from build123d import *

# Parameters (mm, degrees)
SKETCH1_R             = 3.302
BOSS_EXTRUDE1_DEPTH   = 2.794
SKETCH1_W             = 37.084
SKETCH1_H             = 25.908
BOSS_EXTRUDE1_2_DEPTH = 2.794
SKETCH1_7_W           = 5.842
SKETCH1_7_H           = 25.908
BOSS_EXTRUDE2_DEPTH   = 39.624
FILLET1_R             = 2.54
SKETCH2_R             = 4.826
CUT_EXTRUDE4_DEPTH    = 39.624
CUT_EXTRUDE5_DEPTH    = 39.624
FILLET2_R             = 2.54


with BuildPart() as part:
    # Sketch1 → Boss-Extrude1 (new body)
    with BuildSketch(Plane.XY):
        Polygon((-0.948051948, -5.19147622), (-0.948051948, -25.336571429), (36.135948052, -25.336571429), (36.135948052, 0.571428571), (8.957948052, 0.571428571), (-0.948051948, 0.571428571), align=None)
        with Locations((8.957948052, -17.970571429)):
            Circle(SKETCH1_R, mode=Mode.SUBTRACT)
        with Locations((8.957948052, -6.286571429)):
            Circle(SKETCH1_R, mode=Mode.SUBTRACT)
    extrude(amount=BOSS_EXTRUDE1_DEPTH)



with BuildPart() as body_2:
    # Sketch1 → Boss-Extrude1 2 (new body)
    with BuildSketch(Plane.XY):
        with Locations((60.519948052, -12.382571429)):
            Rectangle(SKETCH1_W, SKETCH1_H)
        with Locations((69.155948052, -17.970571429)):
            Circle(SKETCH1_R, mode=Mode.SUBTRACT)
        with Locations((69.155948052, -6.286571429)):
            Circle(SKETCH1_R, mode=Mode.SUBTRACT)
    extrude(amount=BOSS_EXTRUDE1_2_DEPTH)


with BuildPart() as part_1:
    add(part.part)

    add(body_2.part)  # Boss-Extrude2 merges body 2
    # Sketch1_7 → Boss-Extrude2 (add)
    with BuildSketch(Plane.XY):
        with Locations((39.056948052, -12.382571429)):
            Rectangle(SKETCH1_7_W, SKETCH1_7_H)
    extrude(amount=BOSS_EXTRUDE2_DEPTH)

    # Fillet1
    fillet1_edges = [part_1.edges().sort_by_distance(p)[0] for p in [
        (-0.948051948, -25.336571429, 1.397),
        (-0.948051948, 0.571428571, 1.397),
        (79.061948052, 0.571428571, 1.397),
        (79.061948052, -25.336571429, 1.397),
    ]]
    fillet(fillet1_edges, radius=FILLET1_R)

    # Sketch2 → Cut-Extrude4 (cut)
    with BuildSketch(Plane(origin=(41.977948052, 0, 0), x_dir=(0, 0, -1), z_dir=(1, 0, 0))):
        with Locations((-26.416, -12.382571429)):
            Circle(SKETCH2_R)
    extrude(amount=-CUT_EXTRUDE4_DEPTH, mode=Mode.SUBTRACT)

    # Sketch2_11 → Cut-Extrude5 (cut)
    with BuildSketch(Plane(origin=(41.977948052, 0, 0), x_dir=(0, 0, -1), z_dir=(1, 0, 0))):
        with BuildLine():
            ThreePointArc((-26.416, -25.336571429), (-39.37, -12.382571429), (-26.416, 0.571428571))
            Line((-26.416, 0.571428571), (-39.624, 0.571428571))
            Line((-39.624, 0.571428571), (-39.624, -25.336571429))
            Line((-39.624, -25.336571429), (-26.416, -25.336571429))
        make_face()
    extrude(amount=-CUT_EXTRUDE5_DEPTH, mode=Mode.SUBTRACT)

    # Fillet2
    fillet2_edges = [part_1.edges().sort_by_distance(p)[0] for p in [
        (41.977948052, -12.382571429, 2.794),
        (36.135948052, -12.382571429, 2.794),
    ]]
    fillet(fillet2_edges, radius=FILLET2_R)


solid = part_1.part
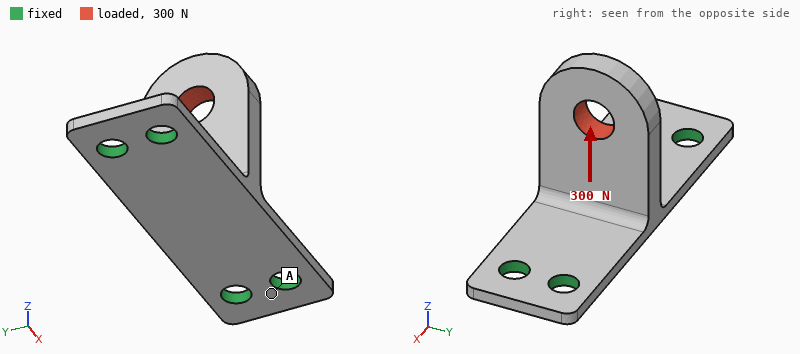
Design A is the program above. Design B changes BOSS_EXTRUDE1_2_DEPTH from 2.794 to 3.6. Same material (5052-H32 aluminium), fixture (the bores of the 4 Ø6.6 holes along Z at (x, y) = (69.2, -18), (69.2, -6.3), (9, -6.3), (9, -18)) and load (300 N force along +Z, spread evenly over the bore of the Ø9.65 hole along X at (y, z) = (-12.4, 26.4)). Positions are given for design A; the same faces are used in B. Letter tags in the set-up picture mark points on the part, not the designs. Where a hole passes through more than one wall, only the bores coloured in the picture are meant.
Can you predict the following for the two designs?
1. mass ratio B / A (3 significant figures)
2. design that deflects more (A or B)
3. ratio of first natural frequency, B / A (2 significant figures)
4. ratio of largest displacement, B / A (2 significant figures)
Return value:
1.07
A
1.2
0.91
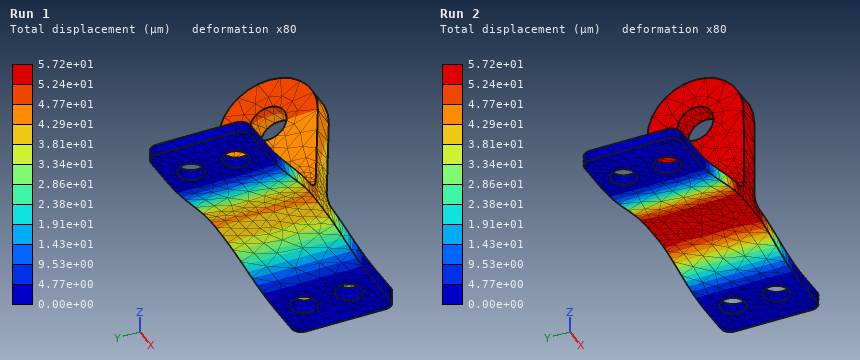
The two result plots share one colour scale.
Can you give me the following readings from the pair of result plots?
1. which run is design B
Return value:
Run 1
